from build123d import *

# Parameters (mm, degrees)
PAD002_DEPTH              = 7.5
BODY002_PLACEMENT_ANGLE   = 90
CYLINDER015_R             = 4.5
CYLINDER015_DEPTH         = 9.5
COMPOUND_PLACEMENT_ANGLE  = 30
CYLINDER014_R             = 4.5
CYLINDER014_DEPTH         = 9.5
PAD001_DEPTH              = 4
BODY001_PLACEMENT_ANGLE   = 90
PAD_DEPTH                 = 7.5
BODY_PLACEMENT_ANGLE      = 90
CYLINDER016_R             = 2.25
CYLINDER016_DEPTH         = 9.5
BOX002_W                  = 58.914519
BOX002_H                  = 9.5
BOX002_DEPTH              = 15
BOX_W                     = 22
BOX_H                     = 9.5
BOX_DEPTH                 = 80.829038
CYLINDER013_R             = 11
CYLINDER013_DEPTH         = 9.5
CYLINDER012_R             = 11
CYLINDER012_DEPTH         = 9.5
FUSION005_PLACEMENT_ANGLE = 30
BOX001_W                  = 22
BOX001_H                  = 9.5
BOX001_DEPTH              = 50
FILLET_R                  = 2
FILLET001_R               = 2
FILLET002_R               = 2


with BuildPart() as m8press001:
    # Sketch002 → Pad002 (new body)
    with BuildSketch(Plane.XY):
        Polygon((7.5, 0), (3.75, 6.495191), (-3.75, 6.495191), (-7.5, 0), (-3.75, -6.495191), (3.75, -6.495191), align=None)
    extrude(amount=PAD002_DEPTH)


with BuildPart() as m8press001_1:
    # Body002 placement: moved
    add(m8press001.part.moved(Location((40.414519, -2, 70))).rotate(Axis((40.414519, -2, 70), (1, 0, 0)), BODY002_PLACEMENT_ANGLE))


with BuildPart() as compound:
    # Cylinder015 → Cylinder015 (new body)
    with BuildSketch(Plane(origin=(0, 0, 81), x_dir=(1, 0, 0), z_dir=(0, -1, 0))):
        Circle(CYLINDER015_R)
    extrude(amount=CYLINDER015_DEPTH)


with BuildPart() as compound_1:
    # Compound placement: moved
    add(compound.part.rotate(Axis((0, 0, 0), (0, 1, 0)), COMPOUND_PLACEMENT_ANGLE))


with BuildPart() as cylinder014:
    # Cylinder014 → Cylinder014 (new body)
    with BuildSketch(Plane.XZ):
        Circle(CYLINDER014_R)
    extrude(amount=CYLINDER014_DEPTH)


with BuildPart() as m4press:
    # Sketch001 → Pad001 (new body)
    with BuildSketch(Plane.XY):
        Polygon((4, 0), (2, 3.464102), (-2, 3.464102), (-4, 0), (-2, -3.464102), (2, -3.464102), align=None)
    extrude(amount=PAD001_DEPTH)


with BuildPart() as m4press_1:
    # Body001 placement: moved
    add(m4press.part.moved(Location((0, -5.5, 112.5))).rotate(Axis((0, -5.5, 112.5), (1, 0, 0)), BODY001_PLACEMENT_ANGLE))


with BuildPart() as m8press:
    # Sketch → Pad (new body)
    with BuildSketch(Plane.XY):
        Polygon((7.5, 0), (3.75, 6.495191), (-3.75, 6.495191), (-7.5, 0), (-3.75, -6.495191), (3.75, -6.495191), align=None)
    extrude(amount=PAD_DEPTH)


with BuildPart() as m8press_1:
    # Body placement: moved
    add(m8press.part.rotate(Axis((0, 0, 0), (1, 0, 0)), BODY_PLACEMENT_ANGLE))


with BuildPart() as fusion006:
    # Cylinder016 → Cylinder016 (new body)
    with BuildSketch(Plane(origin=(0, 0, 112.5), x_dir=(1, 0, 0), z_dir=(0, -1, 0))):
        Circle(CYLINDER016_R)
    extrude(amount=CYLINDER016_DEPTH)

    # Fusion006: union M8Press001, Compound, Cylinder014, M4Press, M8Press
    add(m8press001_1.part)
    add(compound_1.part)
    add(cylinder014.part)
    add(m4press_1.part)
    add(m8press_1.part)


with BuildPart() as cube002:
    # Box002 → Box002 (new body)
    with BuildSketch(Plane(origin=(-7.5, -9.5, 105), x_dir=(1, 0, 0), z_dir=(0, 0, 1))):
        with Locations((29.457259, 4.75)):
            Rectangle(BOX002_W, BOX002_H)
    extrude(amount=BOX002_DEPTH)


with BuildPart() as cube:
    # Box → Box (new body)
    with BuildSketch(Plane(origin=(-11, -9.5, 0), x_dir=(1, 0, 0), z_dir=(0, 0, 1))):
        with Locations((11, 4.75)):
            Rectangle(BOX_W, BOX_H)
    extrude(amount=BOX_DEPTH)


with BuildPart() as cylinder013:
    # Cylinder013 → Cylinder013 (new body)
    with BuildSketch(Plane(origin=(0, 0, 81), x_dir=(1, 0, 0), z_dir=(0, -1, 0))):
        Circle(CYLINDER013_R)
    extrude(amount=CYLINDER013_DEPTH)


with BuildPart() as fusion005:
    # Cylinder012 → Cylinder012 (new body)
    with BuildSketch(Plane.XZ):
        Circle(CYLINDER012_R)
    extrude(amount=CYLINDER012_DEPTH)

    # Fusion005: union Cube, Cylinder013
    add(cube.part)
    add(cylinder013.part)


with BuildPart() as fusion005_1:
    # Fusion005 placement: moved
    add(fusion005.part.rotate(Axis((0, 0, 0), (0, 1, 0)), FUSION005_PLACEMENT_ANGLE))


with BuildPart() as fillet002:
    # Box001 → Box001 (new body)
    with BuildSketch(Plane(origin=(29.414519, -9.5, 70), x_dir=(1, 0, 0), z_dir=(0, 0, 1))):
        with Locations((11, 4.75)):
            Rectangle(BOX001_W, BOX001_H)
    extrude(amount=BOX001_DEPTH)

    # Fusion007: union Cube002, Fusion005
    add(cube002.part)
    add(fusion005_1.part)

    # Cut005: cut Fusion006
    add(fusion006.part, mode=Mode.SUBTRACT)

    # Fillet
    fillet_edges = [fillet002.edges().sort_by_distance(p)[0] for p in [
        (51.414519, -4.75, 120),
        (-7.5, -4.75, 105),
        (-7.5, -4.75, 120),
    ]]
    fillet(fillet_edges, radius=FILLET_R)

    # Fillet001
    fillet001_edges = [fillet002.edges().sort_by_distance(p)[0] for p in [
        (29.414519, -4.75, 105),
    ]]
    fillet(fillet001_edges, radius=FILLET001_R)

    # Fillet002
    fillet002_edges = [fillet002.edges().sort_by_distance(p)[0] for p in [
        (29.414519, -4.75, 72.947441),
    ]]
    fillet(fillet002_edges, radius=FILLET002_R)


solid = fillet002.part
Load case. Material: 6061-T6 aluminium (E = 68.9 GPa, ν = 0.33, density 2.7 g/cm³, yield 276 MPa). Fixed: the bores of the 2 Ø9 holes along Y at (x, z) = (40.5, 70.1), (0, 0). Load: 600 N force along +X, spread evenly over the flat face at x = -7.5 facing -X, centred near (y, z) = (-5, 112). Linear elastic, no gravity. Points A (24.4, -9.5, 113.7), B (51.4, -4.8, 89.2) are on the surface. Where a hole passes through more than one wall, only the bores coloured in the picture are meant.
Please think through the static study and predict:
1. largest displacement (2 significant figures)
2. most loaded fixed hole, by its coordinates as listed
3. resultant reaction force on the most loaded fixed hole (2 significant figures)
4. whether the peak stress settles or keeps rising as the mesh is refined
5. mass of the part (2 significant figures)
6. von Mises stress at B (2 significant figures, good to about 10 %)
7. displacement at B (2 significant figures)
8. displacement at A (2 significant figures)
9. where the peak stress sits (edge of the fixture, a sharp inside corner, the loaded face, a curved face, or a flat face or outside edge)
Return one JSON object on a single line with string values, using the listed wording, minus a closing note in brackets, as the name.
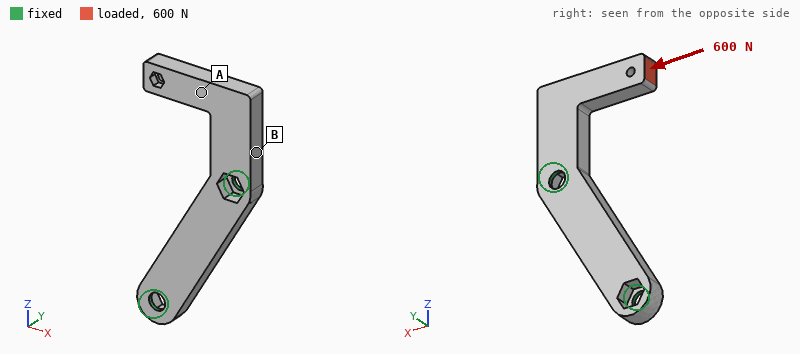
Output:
{"largest displacement": "0.12 mm", "most loaded fixed hole, by its coordinates as listed": "(40.5, 70.1)", "resultant reaction force on the most loaded fixed hole": "720 N", "whether the peak stress settles or keeps rising as the mesh is refined": "keeps rising", "mass of the part": "86 g", "von Mises stress at B": "19 MPa", "displacement at B": "0.030 mm", "displacement at A": "0.075 mm", "where the peak stress sits": "edge of the fixture"}
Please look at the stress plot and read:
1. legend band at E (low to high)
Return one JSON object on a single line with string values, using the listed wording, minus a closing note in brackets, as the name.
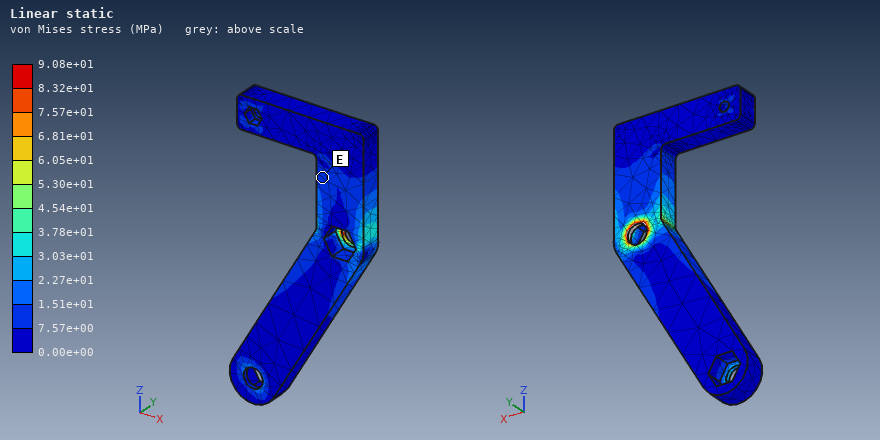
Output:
{"legend band at E": "7.57e+00 to 1.51e+01 MPa"}
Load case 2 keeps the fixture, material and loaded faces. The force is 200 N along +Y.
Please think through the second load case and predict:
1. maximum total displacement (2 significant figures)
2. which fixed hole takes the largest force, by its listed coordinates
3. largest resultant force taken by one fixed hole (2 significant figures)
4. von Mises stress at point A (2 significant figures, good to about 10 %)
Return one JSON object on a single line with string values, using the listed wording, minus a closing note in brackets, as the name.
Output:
{"maximum total displacement": "0.44 mm", "which fixed hole takes the largest force, by its listed coordinates": "(40.5, 70.1)", "largest resultant force taken by one fixed hole": "250 N", "von Mises stress at point A": "27 MPa"}
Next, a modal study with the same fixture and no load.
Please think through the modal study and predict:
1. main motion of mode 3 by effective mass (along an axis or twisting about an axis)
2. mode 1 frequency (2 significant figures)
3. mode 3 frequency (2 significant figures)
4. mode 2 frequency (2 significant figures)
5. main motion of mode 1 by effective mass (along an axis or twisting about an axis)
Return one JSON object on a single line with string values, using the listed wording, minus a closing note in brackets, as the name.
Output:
{"main motion of mode 3 by effective mass": "twisting about Z", "mode 1 frequency": "1200 Hz", "mode 3 frequency": "2800 Hz", "mode 2 frequency": "2500 Hz", "main motion of mode 1 by effective mass": "along Y"}
